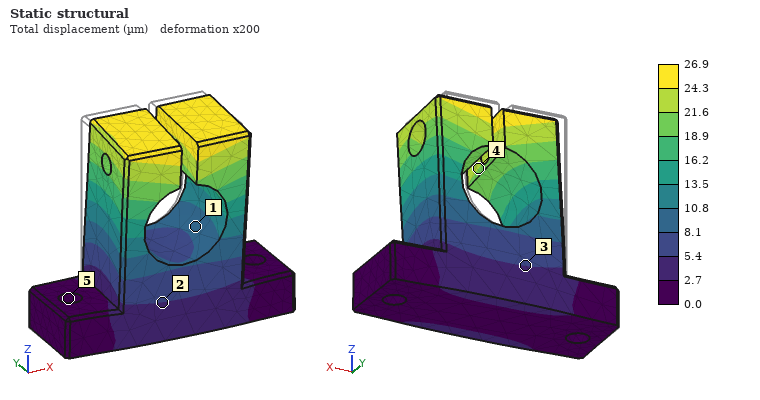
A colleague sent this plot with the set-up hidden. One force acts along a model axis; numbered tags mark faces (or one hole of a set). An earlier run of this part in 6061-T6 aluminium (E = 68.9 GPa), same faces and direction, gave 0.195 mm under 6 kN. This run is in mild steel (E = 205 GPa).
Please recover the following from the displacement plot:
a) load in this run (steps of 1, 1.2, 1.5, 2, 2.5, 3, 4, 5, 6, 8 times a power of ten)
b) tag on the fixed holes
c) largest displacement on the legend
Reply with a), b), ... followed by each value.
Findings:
a) 2.5 kN
b) 5
c) 26.9 µm
